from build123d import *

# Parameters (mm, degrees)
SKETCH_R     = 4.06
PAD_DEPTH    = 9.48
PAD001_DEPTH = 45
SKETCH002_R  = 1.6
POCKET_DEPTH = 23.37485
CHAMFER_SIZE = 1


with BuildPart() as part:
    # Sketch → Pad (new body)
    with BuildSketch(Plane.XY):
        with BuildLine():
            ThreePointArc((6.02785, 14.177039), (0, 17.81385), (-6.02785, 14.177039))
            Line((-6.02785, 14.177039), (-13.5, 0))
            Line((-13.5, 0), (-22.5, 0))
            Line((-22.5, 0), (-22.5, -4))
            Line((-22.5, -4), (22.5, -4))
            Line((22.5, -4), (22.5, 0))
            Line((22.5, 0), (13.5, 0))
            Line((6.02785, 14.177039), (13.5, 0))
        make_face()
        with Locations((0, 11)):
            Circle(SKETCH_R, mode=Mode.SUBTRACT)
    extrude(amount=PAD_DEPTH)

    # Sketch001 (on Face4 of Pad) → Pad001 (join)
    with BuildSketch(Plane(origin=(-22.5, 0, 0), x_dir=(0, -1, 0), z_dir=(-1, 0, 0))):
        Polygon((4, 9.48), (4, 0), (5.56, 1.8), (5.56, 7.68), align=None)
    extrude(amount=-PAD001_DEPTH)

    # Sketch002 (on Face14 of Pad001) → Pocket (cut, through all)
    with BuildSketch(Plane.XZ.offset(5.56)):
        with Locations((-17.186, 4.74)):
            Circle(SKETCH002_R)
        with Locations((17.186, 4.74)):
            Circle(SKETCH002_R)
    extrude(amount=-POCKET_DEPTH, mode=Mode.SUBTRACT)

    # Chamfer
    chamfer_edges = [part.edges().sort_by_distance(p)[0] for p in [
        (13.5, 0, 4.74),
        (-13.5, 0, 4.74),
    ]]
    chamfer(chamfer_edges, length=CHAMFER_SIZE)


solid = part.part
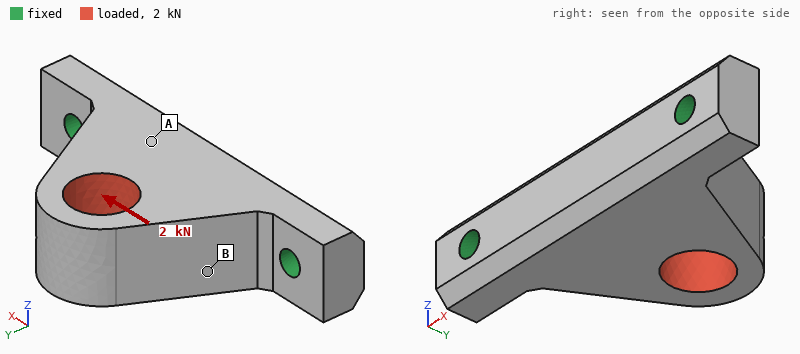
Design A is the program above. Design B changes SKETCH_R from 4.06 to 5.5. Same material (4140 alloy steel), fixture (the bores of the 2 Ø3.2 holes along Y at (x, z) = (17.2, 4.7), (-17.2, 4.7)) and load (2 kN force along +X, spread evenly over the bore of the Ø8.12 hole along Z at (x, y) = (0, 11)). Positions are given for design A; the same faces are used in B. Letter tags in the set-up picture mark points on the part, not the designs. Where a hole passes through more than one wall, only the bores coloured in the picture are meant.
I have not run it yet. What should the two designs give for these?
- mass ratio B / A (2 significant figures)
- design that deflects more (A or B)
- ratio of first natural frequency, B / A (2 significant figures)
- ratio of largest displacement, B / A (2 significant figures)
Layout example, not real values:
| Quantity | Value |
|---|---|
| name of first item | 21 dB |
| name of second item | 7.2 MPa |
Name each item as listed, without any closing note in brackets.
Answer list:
| Quantity | Value |
|---|---|
| mass ratio B / A | 0.91 |
| design that deflects more | B |
| ratio of first natural frequency, B / A | 1.2 |
| ratio of largest displacement, B / A | 2.7 |
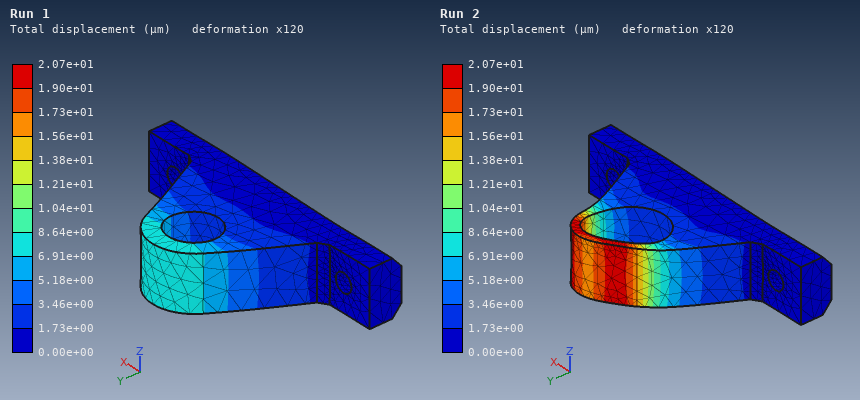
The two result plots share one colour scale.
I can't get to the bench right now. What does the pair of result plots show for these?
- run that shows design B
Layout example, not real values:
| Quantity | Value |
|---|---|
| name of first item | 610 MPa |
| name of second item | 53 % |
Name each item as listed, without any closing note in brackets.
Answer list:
| Quantity | Value |
|---|---|
| run that shows design B | Run 2 |
